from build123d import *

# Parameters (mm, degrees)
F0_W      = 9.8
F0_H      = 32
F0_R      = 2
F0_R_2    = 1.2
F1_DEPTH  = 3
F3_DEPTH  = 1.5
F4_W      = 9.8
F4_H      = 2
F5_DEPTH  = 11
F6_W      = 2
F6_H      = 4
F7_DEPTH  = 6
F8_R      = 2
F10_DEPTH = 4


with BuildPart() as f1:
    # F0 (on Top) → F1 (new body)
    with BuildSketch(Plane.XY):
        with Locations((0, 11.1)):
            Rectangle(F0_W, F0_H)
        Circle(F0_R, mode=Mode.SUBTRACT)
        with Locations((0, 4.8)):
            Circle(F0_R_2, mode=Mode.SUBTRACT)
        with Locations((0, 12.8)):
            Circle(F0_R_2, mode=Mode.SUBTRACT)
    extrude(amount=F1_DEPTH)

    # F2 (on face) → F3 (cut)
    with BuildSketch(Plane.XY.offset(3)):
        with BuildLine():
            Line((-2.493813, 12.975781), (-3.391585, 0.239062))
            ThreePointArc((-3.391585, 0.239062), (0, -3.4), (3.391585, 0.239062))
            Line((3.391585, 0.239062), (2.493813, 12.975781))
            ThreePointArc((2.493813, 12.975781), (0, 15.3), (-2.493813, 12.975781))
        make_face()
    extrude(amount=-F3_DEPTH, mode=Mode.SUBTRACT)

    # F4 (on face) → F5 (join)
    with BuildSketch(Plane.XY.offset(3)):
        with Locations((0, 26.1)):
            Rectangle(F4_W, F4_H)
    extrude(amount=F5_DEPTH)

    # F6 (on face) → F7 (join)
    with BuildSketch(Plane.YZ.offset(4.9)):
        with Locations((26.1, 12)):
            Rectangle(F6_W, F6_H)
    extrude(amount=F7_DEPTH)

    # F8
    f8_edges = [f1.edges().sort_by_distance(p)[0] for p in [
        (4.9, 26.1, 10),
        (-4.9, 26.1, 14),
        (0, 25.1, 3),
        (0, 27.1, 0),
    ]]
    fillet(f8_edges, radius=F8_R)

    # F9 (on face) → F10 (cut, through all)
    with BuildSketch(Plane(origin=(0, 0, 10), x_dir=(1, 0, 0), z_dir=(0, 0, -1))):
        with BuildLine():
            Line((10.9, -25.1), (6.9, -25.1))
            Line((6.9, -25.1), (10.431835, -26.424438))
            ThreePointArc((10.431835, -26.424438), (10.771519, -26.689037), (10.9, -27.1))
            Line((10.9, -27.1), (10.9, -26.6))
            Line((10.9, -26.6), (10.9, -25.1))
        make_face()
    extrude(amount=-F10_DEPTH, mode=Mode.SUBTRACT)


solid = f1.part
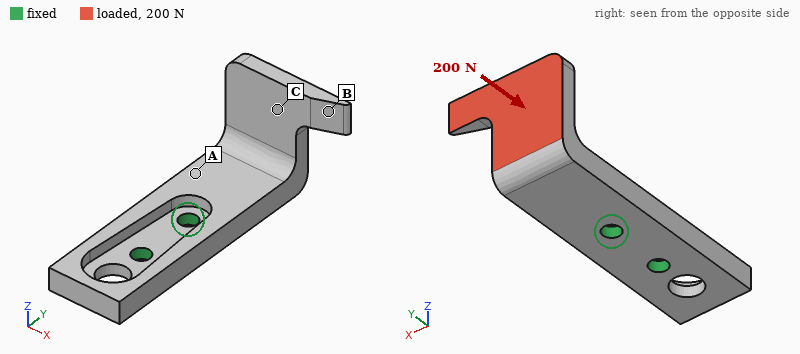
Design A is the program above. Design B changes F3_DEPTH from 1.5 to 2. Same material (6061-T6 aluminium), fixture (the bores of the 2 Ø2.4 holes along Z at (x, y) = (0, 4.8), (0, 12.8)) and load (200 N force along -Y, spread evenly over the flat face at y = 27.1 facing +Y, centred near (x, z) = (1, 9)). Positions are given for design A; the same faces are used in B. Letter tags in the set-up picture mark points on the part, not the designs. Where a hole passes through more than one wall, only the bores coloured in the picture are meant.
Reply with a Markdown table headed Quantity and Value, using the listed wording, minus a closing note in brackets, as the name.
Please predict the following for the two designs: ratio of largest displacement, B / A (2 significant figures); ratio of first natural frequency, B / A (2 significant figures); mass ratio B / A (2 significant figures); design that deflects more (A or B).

| Quantity | Value |
|---|---|
| ratio of largest displacement, B / A | 1.1 |
| ratio of first natural frequency, B / A | 0.92 |
| mass ratio B / A | 0.96 |
| design that deflects more | B |
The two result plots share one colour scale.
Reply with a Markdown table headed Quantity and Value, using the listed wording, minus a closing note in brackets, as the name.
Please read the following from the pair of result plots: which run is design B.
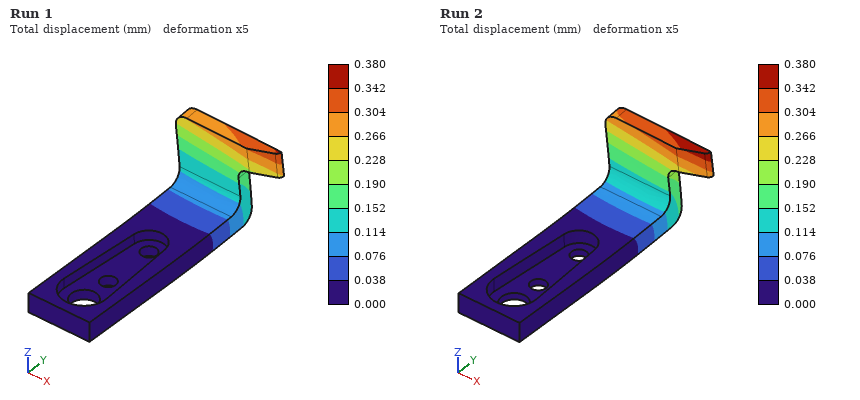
| Quantity | Value |
|---|---|
| which run is design B | Run 2 |
